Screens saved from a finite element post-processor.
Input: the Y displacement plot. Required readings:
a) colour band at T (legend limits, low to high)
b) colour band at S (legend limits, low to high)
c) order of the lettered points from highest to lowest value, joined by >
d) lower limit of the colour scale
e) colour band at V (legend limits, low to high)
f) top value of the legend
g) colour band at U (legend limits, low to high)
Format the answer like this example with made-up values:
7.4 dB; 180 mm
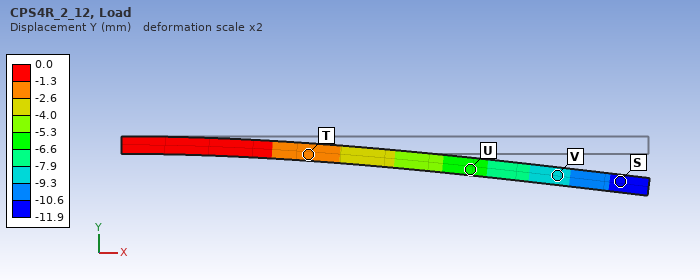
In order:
-2.6 to -1.3 mm; -11.9 to -10.6 mm; T > U > V > S; -11.9 mm; -9.3 to -7.9 mm; 0.0 mm; -6.6 to -5.3 mm
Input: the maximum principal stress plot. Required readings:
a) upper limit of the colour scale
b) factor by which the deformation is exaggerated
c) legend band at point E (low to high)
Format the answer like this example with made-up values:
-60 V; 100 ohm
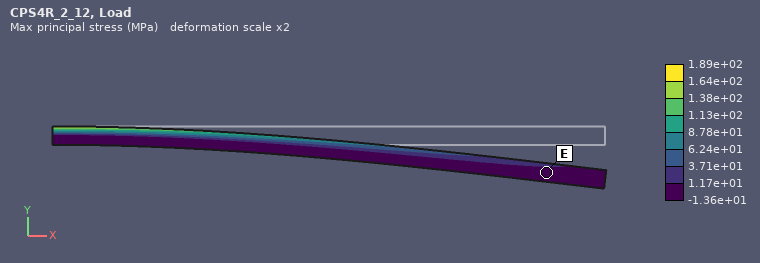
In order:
1.89e+02 MPa; 2; -1.36e+01 to 1.17e+01 MPa
